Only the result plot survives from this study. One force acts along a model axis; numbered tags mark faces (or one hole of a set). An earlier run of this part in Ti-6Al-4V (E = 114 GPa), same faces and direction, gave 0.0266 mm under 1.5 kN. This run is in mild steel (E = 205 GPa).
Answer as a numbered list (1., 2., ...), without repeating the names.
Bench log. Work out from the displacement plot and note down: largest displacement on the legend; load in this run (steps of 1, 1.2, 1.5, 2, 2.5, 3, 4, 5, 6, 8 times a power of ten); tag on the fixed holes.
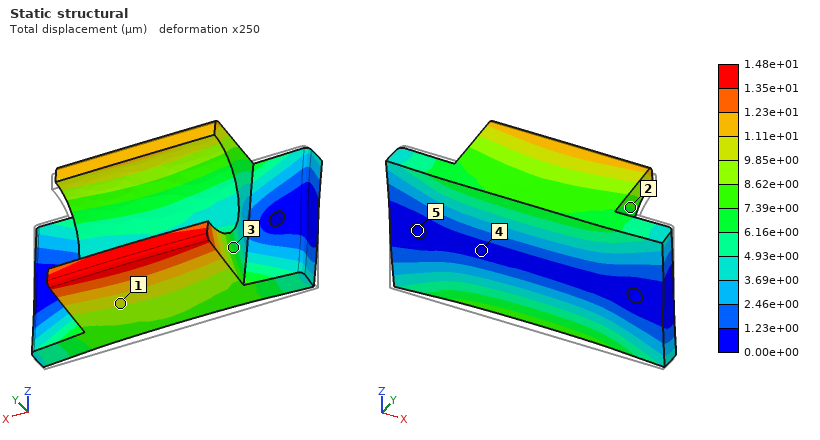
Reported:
1. 1.48e+01 µm
2. 1.5 kN
3. 5
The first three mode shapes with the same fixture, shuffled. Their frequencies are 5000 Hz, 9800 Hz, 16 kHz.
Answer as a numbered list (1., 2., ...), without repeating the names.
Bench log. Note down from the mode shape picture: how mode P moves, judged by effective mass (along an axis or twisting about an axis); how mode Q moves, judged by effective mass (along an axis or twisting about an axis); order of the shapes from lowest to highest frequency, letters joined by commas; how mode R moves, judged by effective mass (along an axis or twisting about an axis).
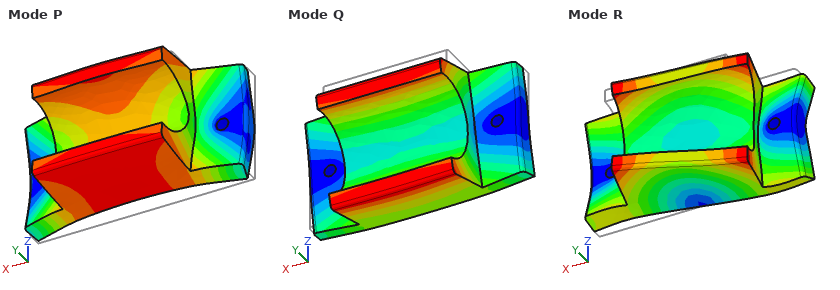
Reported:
1. along Y
2. along Z
3. Q, P, R
4. along X
